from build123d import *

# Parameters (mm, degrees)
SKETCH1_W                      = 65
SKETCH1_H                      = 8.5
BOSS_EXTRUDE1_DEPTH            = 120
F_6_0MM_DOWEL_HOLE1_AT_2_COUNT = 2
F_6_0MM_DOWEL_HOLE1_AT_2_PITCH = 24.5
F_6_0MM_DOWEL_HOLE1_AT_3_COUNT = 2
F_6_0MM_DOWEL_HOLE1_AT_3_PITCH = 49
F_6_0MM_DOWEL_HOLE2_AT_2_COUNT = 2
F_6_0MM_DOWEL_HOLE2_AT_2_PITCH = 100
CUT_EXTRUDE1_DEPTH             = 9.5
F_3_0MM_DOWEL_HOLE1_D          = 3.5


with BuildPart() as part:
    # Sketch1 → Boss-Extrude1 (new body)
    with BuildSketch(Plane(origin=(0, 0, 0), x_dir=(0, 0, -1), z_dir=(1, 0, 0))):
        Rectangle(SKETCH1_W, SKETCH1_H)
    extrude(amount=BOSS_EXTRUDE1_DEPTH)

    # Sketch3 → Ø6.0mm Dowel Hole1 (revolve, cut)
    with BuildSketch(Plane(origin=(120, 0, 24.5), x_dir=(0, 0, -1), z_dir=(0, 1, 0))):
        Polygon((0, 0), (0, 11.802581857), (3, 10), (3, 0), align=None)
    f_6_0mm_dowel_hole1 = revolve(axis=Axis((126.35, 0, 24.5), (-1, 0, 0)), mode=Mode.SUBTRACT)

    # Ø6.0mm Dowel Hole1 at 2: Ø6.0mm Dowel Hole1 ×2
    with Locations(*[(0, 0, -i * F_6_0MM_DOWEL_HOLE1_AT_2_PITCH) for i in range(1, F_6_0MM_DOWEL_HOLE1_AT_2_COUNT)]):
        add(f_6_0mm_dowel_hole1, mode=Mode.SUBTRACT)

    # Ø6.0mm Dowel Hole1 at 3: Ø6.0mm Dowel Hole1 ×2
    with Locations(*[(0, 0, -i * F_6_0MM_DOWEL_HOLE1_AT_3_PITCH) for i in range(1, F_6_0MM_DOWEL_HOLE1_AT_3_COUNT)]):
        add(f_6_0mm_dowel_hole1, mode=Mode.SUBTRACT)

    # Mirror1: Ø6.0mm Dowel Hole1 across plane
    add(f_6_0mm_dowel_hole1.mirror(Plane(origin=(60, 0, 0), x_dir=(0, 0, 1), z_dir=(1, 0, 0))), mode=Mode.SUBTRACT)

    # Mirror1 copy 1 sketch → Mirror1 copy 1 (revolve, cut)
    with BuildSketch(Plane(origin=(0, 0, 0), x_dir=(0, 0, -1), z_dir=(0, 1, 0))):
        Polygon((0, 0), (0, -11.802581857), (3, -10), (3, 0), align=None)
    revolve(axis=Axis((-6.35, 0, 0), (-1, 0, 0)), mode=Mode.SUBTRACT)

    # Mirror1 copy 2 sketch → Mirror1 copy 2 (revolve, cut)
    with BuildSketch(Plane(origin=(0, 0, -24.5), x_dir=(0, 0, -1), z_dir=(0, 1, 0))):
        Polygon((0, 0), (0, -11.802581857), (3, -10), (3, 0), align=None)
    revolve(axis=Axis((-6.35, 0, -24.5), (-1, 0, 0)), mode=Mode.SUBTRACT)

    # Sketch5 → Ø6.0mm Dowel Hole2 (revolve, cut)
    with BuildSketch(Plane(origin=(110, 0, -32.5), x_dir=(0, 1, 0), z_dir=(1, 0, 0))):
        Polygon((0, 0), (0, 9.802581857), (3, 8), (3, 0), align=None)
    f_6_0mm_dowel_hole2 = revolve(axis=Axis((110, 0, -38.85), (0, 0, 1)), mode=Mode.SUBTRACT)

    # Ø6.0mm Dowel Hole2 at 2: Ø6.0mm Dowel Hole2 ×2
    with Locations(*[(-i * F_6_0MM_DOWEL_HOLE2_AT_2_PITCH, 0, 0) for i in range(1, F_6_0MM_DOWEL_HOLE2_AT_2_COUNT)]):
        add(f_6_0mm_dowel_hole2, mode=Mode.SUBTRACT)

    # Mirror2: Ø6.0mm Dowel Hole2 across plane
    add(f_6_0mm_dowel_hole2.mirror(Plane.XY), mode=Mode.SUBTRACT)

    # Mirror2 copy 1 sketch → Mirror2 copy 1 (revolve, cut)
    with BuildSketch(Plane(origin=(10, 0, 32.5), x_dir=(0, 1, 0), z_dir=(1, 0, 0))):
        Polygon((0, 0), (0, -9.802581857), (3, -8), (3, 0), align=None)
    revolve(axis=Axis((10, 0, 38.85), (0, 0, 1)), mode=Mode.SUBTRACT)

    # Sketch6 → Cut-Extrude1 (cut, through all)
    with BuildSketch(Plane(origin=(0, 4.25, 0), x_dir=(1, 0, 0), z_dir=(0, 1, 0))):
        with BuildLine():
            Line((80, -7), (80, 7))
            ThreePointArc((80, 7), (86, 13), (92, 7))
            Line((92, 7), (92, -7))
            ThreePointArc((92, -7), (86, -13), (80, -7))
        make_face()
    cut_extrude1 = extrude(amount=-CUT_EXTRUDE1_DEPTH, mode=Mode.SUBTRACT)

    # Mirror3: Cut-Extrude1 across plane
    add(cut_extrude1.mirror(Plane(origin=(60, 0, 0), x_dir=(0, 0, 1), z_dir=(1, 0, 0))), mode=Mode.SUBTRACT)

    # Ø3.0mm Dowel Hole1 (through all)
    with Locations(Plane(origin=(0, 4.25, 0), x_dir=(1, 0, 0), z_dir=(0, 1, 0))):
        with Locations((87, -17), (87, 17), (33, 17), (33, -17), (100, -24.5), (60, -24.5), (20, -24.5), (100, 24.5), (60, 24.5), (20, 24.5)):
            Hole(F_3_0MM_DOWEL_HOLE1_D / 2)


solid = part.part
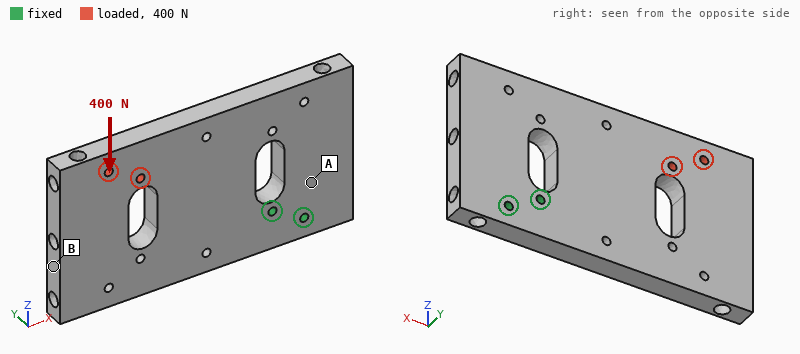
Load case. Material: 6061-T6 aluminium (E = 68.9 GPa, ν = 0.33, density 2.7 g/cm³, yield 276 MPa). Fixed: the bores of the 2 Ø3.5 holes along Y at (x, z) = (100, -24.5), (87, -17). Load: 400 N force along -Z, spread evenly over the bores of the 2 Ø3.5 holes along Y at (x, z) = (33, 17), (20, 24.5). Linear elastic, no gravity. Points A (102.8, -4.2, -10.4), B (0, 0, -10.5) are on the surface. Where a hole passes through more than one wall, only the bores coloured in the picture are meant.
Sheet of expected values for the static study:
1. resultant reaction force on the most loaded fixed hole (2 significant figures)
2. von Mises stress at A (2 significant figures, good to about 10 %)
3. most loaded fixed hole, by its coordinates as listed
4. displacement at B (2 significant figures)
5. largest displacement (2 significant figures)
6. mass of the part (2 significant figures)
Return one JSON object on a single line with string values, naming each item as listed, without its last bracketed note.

{"resultant reaction force on the most loaded fixed hole": "1.7 kN", "von Mises stress at A": "6.6 MPa", "most loaded fixed hole, by its coordinates as listed": "(87, -17)", "displacement at B": "43 µm", "largest displacement": "49 µm", "mass of the part": "160 g"}
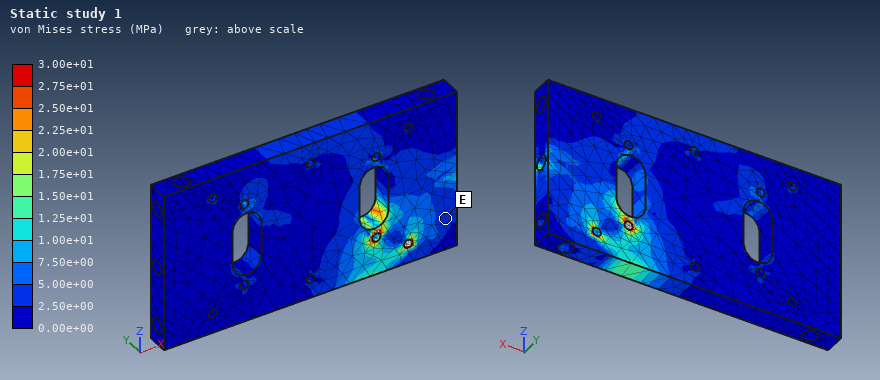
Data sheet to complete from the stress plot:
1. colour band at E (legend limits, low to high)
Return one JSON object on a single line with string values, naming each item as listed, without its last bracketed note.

{"colour band at E": "2.50e+00 to 5.00e+00 MPa"}
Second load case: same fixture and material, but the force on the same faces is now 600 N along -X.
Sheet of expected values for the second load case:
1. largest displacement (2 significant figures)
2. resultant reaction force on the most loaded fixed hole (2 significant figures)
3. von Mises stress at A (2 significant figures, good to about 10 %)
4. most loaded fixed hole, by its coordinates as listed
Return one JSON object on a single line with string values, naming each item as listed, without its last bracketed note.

{"largest displacement": "46 µm", "resultant reaction force on the most loaded fixed hole": "1.7 kN", "von Mises stress at A": "7.5 MPa", "most loaded fixed hole, by its coordinates as listed": "(87, -17)"}
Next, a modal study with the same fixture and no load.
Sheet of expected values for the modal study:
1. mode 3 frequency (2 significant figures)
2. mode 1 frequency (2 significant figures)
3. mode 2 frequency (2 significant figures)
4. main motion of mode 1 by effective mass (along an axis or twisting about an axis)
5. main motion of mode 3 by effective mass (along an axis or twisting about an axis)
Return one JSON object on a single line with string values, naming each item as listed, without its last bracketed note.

{"mode 3 frequency": "1800 Hz", "mode 1 frequency": "670 Hz", "mode 2 frequency": "1500 Hz", "main motion of mode 1 by effective mass": "along Y", "main motion of mode 3 by effective mass": "along Z"}
